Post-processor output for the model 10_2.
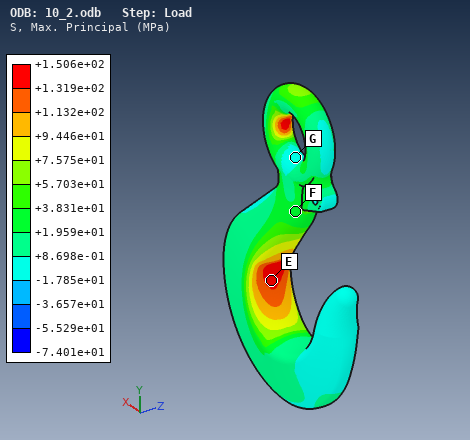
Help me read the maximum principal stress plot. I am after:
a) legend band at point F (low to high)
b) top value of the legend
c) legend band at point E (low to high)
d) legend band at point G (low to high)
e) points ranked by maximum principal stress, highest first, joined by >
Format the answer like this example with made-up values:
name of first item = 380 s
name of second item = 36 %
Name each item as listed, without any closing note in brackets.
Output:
legend band at point F = +1.959e+01 to +3.831e+01 MPa
top value of the legend = +1.506e+02 MPa
legend band at point E = +1.319e+02 to +1.506e+02 MPa
legend band at point G = -1.785e+01 to +8.698e-01 MPa
points ranked by maximum principal stress, highest first, joined by > = E > F > G
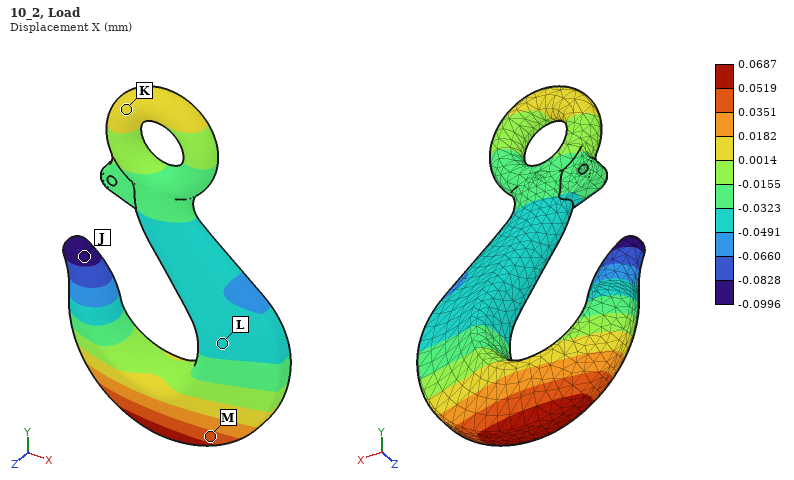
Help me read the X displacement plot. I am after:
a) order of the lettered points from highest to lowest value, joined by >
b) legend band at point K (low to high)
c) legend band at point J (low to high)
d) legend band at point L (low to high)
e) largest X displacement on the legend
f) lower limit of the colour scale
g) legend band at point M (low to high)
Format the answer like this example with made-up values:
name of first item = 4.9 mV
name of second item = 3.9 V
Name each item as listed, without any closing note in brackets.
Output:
order of the lettered points from highest to lowest value, joined by > = M > K > L > J
legend band at point K = 0.0014 to 0.0182 mm
legend band at point J = -0.0996 to -0.0828 mm
legend band at point L = -0.0491 to -0.0323 mm
largest X displacement on the legend = 0.0687 mm
lower limit of the colour scale = -0.0996 mm
legend band at point M = 0.0351 to 0.0519 mm
